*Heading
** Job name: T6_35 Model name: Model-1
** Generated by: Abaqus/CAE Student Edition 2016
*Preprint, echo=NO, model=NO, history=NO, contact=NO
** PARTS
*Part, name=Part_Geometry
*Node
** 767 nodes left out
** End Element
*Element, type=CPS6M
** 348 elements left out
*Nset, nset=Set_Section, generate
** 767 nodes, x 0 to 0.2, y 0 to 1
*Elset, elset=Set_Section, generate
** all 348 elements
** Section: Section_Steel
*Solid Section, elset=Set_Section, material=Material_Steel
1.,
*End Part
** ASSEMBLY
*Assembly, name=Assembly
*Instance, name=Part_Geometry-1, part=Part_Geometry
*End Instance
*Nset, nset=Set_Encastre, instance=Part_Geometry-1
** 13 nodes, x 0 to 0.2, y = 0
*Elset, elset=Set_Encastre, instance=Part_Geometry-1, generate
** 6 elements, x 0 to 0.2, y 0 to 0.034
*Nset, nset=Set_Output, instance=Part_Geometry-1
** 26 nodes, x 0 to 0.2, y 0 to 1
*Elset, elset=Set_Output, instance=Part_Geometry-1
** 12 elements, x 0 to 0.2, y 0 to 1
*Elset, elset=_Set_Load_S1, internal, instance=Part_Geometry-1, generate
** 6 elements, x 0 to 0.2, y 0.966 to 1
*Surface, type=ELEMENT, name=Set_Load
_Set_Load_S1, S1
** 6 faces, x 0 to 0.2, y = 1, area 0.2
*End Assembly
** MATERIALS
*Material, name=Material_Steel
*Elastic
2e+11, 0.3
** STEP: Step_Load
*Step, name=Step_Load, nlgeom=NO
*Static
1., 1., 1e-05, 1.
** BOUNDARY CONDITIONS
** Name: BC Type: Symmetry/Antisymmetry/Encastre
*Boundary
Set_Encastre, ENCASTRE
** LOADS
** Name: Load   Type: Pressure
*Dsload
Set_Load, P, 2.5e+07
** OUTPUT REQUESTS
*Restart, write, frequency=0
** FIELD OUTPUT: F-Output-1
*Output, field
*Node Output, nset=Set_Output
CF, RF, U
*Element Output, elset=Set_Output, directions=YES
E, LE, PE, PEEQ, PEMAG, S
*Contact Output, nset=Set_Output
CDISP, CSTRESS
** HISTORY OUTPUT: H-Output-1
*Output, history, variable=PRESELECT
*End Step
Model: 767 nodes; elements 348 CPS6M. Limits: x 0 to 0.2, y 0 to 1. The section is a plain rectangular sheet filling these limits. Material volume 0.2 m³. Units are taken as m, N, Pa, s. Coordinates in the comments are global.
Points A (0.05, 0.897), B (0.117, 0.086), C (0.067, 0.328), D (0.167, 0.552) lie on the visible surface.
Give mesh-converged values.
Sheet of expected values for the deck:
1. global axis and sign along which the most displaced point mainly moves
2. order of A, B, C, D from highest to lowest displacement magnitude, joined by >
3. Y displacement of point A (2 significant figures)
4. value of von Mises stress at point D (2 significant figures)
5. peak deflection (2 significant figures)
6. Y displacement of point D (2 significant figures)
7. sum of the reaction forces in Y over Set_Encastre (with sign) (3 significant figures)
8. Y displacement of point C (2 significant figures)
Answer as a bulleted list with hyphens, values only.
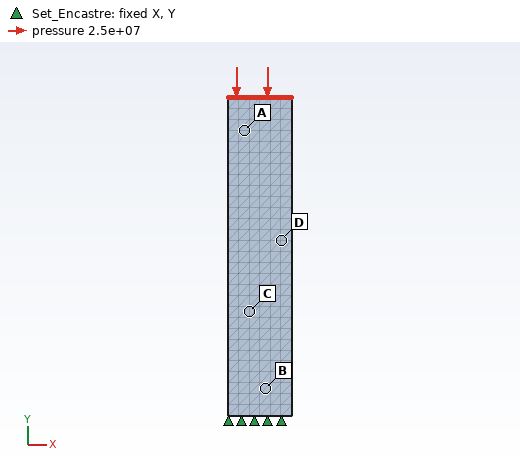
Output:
- -Y
- A > D > C > B
- -1.1e-04 m
- 2.5e+07 Pa
- 1.2e-04 m
- -6.9e-05 m
- 5.00e+06 N
- -4.1e-05 m
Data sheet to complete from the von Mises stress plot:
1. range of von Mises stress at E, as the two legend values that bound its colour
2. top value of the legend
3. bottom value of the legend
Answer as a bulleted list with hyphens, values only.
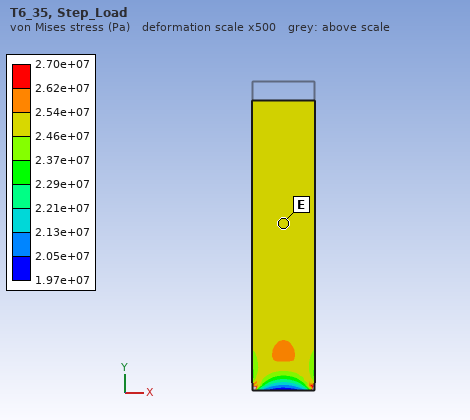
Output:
- 2.46e+07 to 2.54e+07 Pa
- 2.70e+07 Pa
- 1.97e+07 Pa
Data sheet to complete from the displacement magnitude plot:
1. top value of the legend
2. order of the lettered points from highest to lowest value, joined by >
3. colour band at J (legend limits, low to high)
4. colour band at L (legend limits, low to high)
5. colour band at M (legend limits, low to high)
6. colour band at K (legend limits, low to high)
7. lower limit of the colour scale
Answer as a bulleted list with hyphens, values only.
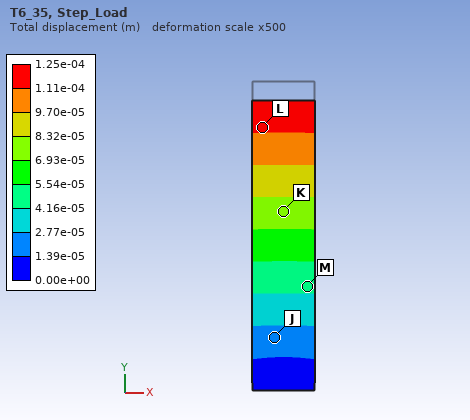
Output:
- 1.25e-04 m
- L > K > M > J
- 1.39e-05 to 2.77e-05 m
- 1.11e-04 to 1.25e-04 m
- 4.16e-05 to 5.54e-05 m
- 6.93e-05 to 8.32e-05 m
- 0.00e+00 m
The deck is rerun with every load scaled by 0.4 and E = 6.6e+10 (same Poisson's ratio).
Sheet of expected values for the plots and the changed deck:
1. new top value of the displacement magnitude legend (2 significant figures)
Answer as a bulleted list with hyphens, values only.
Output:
- 1.5e-04 m
